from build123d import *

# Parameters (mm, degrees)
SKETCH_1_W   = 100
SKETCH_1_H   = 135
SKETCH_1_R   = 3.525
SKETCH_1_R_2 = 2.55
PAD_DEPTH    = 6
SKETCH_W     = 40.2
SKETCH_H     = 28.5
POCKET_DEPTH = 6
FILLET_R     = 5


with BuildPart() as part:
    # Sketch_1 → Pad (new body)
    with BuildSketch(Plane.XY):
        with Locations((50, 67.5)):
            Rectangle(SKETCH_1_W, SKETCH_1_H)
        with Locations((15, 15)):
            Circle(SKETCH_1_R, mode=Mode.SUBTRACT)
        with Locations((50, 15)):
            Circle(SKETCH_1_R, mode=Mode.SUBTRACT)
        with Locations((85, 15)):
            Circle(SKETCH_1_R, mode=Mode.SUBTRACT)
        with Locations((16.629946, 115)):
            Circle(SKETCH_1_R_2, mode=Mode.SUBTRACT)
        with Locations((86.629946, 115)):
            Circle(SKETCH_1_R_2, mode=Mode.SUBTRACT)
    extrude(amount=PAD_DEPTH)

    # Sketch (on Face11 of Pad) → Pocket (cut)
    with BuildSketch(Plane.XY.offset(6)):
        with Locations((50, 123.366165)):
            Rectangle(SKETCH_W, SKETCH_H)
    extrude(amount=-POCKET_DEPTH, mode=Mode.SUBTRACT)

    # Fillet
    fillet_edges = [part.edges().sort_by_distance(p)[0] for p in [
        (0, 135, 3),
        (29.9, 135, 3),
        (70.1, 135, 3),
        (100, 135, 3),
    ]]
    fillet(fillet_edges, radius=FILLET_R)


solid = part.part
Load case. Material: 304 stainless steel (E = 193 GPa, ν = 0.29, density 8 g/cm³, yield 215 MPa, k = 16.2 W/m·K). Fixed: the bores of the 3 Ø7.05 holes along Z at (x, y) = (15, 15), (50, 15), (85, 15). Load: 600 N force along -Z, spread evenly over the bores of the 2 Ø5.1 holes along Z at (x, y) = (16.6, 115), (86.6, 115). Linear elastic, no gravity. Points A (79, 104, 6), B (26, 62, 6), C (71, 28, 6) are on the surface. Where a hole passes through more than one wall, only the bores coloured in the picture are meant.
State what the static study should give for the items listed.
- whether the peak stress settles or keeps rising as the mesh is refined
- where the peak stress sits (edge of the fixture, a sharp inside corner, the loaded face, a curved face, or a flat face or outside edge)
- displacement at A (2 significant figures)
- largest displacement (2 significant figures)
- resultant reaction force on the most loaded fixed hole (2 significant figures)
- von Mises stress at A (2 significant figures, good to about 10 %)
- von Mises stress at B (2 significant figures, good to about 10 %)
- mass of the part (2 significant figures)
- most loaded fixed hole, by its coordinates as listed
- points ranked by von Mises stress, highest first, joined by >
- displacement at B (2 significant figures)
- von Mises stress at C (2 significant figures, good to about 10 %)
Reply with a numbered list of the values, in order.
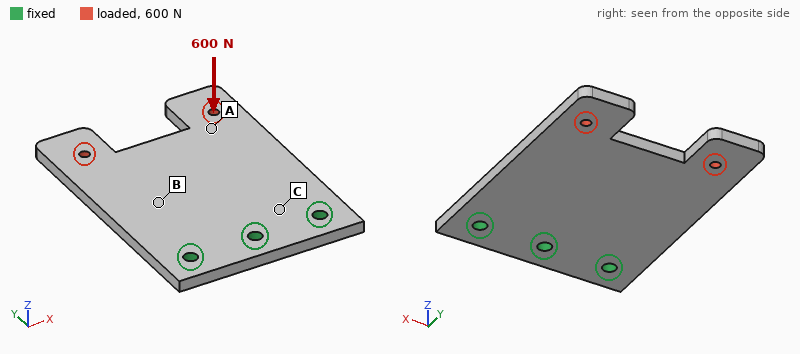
1. keeps rising
2. edge of the fixture
3. 0.46 mm
4. 0.73 mm
5. 350 N
6. 20 MPa
7. 49 MPa
8. 590 g
9. (50, 15)
10. C > B > A
11. 0.15 mm
12. 78 MPa
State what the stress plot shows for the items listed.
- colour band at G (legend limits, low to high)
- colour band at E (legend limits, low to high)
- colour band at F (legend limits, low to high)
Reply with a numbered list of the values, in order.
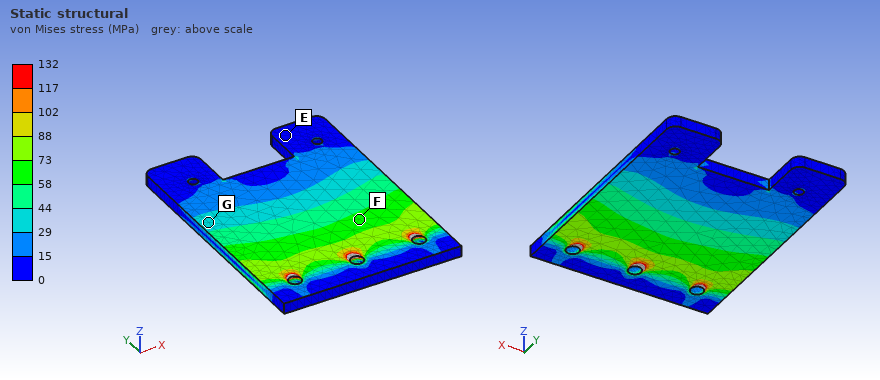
1. 29 to 44 MPa
2. 0 to 15 MPa
3. 58 to 73 MPa
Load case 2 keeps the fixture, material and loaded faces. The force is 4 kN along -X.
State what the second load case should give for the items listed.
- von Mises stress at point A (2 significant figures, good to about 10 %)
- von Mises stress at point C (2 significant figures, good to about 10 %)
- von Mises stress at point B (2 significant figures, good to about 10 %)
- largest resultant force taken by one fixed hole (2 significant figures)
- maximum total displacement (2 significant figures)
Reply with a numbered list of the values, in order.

1. 17 MPa
2. 22 MPa
3. 16 MPa
4. 5.6 kN
5. 41 µm
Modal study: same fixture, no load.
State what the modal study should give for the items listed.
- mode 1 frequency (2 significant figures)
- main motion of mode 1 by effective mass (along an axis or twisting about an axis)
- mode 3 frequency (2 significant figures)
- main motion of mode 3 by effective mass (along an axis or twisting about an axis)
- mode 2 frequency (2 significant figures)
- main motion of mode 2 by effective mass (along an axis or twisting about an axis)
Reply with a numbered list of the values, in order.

1. 390 Hz
2. along Z
3. 2200 Hz
4. along Z
5. 880 Hz
6. twisting about Y
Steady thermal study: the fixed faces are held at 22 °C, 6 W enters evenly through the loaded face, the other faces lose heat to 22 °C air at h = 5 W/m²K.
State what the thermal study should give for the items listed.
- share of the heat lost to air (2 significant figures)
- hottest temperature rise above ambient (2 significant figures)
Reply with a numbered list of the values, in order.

1. 46 %
2. 53 K
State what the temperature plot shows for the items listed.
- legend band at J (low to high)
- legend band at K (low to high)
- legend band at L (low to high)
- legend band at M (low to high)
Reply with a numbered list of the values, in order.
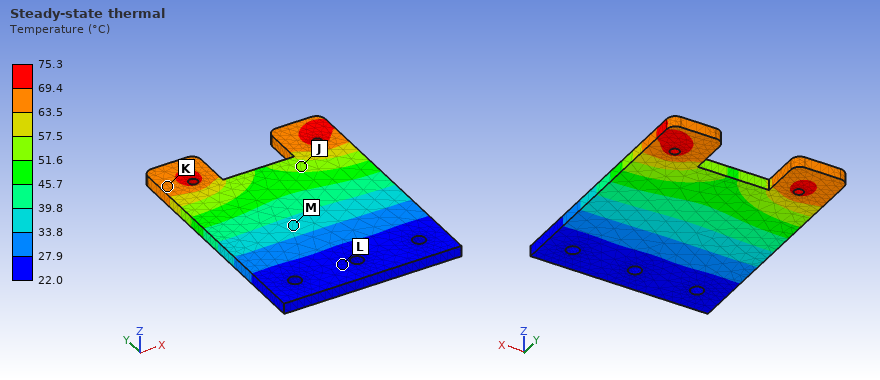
1. 51.6 to 57.5 °C
2. 63.5 to 69.4 °C
3. 22.0 to 27.9 °C
4. 33.8 to 39.8 °C
